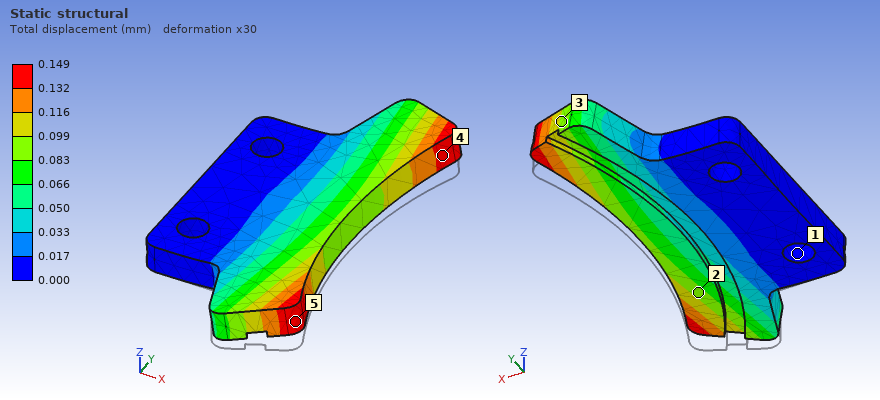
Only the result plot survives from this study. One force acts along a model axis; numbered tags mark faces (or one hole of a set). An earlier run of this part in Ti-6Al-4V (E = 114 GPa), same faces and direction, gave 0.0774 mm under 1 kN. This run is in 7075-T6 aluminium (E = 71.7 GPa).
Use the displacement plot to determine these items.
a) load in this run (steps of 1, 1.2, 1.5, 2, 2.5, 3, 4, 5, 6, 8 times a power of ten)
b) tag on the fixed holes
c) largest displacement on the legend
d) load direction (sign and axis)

1.2 kN
1
0.149 mm
+Z
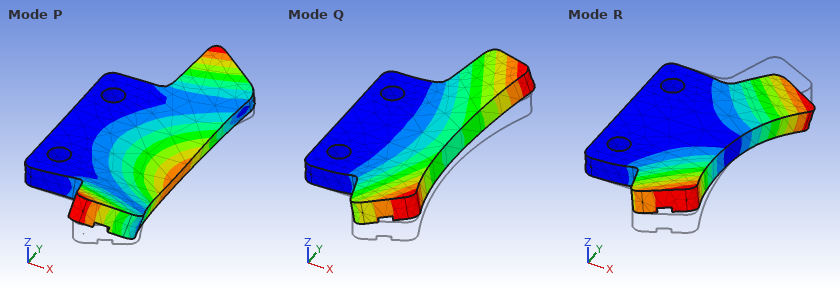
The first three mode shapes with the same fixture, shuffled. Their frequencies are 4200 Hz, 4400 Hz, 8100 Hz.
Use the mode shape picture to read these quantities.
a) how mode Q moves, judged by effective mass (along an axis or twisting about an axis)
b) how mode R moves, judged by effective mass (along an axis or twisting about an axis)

along Z
twisting about X
